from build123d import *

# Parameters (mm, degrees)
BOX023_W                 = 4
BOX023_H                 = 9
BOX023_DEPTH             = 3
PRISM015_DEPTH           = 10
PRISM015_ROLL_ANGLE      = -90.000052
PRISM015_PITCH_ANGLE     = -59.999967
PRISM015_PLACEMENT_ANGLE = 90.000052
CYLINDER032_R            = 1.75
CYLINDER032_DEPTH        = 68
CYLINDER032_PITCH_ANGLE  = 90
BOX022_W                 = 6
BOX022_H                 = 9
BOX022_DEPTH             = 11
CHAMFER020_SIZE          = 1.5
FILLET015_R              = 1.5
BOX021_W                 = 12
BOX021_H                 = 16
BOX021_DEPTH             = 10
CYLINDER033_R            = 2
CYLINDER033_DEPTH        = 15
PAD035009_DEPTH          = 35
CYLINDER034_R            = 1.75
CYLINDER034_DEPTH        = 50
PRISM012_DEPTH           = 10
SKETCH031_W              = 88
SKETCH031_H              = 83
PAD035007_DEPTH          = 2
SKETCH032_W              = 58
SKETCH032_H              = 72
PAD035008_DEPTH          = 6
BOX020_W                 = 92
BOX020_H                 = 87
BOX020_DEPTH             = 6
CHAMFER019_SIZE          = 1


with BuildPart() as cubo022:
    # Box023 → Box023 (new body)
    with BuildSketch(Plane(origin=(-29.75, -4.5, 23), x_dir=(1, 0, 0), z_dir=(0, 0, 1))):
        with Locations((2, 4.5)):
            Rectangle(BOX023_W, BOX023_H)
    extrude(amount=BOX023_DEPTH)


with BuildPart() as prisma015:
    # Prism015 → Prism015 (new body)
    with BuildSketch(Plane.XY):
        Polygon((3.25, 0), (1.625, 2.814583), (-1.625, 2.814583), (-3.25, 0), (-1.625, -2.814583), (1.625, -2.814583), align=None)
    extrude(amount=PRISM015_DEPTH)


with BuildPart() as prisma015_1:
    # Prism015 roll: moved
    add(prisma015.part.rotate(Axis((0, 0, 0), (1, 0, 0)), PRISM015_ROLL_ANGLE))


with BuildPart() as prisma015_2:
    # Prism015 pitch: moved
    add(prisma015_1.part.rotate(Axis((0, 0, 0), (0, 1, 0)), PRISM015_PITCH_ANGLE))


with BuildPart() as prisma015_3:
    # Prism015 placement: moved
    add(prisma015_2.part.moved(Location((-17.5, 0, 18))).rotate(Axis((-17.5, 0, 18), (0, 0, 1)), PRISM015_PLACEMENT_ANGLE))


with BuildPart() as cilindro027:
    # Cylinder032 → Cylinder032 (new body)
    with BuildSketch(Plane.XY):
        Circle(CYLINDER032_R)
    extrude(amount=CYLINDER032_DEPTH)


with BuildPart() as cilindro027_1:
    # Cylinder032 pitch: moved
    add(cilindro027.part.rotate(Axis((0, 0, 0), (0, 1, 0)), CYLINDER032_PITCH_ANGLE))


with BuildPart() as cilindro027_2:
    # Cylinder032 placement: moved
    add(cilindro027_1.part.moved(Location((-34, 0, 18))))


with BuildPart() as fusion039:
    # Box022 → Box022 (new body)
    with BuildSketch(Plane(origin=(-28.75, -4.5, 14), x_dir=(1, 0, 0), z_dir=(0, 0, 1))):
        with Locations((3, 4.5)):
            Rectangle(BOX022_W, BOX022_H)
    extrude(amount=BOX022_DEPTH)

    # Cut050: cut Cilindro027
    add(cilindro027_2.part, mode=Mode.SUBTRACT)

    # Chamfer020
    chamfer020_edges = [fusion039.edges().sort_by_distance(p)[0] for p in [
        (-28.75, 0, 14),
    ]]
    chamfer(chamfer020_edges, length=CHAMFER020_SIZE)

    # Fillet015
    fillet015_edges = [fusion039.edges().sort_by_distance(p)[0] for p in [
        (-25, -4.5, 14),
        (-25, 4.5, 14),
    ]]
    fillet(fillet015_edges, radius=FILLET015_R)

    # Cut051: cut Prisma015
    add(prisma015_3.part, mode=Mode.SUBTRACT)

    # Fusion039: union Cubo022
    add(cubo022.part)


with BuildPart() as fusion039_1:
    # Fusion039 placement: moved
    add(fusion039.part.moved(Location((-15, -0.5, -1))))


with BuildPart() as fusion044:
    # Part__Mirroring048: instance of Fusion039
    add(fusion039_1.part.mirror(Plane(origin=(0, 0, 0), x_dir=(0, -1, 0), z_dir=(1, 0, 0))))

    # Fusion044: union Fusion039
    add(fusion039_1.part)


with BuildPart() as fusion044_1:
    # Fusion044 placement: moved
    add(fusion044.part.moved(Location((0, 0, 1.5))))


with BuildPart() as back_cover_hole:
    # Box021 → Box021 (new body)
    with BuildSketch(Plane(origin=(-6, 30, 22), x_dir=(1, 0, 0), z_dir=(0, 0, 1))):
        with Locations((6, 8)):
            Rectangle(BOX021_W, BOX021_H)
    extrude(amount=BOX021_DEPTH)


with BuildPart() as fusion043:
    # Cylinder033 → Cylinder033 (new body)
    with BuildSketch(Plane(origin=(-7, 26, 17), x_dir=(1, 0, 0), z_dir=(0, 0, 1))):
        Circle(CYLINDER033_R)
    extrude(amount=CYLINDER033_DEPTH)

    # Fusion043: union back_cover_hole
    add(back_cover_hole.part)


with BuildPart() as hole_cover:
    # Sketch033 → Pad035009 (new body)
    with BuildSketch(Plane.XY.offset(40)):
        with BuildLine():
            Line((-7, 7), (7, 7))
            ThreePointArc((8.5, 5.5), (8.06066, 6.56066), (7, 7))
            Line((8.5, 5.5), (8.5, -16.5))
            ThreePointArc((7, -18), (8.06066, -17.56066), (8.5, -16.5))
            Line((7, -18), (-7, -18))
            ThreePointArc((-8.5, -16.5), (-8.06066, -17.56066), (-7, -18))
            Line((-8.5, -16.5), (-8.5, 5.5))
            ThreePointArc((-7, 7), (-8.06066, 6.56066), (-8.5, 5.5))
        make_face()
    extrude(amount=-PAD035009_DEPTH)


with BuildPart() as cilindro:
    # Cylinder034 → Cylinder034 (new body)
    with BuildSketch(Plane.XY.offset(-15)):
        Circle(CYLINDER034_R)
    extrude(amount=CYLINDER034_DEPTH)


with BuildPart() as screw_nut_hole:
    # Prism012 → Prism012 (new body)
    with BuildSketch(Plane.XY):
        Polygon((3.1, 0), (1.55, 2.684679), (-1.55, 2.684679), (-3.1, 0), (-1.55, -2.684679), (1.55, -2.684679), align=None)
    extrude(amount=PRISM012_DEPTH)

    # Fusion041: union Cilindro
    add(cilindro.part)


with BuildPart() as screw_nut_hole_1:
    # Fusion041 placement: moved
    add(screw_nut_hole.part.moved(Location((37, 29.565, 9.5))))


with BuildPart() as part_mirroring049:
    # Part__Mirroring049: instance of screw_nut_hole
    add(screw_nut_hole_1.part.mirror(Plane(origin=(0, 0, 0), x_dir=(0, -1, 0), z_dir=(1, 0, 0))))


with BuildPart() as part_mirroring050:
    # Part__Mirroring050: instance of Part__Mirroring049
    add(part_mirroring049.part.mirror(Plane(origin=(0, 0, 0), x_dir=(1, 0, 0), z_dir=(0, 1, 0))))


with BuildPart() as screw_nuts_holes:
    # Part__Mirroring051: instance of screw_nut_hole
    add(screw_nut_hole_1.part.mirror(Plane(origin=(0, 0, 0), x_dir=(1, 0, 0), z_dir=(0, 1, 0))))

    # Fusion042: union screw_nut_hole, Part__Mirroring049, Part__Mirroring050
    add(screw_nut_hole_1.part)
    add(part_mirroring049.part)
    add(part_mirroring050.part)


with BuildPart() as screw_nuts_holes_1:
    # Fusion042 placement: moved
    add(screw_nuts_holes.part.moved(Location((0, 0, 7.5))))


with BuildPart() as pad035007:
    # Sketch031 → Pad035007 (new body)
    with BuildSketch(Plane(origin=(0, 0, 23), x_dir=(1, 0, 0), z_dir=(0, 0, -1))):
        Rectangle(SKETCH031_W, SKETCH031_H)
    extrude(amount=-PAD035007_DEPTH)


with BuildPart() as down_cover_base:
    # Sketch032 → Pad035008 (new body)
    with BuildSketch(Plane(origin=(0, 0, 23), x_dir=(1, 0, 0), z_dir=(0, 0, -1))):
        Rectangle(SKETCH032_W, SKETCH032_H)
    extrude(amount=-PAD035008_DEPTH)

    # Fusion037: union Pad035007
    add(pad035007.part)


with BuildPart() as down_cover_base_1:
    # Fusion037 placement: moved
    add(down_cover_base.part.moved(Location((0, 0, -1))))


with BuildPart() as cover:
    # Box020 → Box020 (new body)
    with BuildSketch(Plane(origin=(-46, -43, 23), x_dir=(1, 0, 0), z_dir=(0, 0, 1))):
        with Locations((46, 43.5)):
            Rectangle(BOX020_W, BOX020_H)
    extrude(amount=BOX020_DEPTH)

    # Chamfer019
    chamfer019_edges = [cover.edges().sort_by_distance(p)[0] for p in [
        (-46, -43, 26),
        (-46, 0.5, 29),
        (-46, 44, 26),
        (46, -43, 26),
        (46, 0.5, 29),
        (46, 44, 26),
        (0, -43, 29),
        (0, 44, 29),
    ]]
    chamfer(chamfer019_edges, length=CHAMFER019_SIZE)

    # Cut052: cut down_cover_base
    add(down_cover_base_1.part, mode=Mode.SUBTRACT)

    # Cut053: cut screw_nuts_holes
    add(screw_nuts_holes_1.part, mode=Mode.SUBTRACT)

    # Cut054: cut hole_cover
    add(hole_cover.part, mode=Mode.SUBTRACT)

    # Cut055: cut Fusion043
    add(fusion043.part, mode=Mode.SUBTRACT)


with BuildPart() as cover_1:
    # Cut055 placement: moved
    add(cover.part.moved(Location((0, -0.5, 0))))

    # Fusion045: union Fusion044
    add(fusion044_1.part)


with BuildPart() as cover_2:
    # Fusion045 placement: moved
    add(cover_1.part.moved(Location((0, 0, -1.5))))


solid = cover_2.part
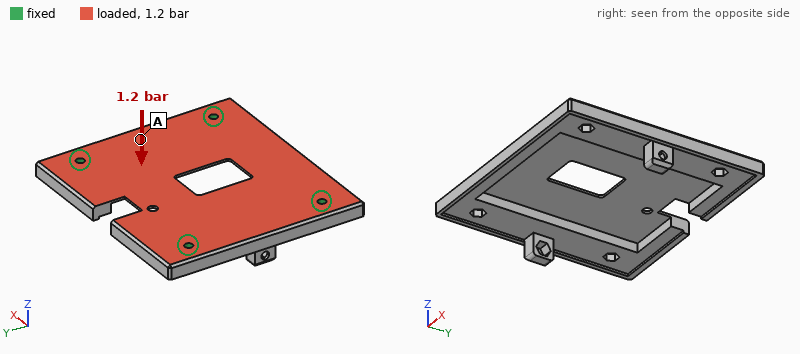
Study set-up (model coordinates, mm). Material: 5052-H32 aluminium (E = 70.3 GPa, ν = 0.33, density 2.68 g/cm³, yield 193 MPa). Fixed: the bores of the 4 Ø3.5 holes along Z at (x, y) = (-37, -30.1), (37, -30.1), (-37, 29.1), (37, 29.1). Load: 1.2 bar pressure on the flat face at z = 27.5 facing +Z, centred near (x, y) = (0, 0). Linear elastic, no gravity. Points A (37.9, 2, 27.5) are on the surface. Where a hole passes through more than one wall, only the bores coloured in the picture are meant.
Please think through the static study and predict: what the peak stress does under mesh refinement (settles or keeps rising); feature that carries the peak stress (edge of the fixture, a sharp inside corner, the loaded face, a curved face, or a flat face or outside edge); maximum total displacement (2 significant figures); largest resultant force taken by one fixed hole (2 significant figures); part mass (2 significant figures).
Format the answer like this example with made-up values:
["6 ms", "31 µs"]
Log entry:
["keeps rising", "edge of the fixture", "0.49 mm", "280 N", "62 g"]
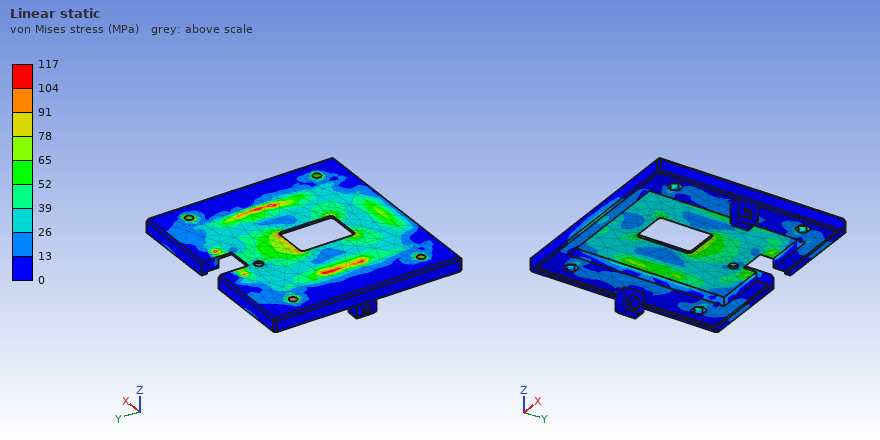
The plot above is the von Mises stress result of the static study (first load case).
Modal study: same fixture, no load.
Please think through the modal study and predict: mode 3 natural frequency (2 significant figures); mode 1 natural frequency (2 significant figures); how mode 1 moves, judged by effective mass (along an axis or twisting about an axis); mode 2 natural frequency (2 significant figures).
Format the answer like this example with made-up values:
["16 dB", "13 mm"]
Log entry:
["3300 Hz", "2100 Hz", "along Z", "3000 Hz"]
